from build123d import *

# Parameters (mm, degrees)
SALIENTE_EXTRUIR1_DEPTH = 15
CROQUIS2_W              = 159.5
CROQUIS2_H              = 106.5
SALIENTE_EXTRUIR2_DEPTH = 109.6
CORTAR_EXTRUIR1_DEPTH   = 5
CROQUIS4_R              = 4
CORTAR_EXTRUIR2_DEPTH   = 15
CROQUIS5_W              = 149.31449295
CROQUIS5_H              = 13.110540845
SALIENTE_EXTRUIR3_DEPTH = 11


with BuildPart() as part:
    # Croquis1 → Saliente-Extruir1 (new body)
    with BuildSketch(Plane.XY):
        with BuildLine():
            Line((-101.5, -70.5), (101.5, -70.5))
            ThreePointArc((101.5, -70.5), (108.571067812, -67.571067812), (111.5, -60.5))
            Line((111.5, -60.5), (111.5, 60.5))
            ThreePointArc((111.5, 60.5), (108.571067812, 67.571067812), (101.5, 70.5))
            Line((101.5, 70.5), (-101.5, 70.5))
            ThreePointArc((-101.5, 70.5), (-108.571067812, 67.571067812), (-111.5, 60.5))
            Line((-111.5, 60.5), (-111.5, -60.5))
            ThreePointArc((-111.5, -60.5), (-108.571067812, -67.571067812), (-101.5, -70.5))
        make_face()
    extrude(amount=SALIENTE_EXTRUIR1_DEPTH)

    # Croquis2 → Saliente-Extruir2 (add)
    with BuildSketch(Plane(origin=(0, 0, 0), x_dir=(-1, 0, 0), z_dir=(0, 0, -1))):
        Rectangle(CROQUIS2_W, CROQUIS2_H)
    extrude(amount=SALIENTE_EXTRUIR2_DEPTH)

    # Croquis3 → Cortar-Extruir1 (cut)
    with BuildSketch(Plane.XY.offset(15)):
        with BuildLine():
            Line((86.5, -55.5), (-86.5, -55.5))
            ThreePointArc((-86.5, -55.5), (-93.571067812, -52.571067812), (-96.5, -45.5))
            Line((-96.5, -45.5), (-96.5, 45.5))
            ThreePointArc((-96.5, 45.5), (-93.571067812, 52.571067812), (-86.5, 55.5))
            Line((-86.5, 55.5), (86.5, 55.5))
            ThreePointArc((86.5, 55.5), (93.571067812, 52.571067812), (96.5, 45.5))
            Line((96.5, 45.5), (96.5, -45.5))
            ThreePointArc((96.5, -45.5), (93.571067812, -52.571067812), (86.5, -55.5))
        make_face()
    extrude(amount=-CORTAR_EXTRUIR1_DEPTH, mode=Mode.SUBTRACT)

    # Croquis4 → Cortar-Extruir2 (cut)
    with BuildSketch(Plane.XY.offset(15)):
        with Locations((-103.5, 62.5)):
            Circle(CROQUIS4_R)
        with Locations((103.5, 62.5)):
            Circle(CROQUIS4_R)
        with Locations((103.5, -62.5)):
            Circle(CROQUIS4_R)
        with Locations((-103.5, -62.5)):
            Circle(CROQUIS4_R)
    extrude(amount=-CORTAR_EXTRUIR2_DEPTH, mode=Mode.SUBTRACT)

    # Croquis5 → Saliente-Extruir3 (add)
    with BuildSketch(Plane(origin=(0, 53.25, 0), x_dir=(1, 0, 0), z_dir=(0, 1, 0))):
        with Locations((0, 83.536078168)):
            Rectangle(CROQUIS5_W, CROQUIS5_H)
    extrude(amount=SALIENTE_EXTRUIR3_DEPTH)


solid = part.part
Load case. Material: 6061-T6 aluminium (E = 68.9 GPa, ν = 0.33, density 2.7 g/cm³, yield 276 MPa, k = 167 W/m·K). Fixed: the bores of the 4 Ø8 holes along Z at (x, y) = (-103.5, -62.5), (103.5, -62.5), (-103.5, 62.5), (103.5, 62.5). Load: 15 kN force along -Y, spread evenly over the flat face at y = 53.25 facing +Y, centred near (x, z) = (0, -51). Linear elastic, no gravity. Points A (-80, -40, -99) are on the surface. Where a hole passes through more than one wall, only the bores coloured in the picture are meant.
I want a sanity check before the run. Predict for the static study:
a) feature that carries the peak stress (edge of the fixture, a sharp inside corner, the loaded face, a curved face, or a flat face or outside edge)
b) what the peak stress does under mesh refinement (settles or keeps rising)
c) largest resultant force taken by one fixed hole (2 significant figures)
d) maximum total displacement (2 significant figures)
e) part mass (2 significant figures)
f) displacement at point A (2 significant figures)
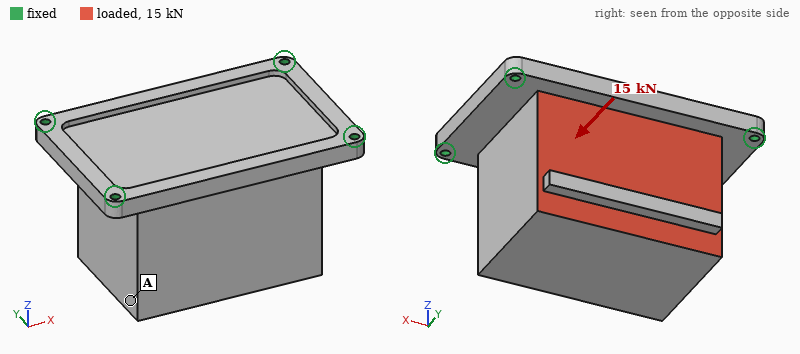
edge of the fixture
keeps rising
6.3 kN
0.11 mm
6.1 kg
0.100 mm
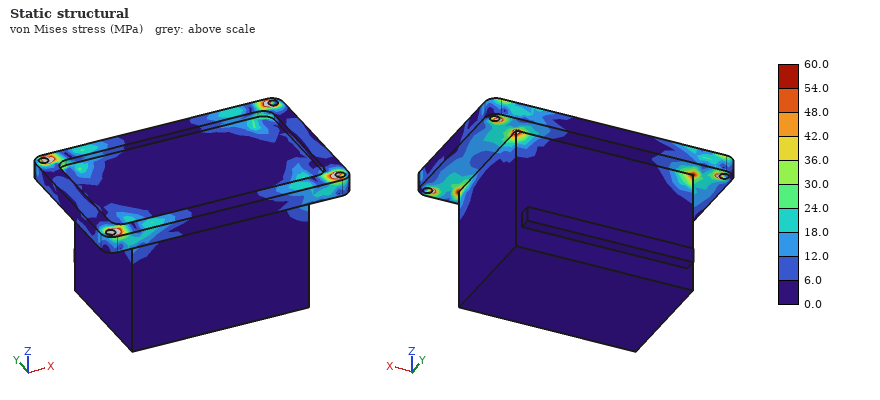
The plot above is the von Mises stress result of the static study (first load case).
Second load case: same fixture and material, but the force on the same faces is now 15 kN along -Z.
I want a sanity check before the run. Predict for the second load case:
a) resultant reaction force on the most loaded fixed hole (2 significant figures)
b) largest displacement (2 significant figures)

8.1 kN
0.13 mm
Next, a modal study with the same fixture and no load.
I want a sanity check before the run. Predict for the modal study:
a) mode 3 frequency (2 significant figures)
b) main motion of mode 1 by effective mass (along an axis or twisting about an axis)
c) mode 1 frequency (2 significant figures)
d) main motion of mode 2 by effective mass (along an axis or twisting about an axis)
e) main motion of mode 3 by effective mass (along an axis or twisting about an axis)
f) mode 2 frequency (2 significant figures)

1300 Hz
along Y
900 Hz
along Z
along X
1200 Hz
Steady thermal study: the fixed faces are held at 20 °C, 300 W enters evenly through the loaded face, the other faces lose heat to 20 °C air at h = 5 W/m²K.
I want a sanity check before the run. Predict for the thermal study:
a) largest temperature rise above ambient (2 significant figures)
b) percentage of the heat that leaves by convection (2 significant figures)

42 K
6.4 %
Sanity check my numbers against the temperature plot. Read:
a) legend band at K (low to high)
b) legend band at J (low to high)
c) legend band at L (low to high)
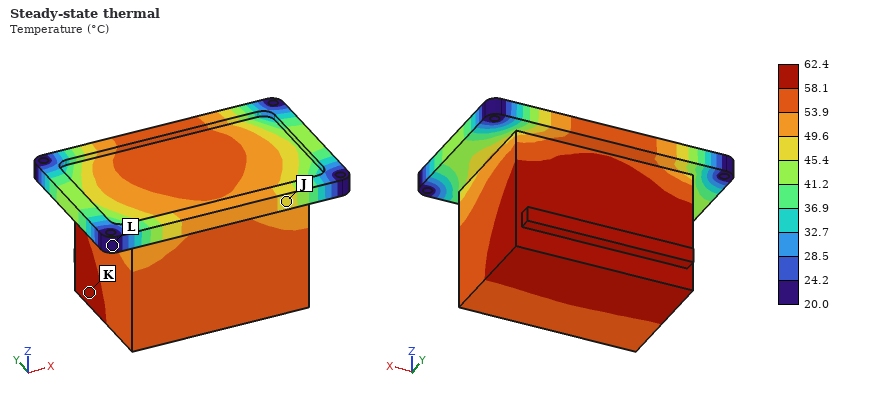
58.1 to 62.4 °C
45.4 to 49.6 °C
20.0 to 24.2 °C
